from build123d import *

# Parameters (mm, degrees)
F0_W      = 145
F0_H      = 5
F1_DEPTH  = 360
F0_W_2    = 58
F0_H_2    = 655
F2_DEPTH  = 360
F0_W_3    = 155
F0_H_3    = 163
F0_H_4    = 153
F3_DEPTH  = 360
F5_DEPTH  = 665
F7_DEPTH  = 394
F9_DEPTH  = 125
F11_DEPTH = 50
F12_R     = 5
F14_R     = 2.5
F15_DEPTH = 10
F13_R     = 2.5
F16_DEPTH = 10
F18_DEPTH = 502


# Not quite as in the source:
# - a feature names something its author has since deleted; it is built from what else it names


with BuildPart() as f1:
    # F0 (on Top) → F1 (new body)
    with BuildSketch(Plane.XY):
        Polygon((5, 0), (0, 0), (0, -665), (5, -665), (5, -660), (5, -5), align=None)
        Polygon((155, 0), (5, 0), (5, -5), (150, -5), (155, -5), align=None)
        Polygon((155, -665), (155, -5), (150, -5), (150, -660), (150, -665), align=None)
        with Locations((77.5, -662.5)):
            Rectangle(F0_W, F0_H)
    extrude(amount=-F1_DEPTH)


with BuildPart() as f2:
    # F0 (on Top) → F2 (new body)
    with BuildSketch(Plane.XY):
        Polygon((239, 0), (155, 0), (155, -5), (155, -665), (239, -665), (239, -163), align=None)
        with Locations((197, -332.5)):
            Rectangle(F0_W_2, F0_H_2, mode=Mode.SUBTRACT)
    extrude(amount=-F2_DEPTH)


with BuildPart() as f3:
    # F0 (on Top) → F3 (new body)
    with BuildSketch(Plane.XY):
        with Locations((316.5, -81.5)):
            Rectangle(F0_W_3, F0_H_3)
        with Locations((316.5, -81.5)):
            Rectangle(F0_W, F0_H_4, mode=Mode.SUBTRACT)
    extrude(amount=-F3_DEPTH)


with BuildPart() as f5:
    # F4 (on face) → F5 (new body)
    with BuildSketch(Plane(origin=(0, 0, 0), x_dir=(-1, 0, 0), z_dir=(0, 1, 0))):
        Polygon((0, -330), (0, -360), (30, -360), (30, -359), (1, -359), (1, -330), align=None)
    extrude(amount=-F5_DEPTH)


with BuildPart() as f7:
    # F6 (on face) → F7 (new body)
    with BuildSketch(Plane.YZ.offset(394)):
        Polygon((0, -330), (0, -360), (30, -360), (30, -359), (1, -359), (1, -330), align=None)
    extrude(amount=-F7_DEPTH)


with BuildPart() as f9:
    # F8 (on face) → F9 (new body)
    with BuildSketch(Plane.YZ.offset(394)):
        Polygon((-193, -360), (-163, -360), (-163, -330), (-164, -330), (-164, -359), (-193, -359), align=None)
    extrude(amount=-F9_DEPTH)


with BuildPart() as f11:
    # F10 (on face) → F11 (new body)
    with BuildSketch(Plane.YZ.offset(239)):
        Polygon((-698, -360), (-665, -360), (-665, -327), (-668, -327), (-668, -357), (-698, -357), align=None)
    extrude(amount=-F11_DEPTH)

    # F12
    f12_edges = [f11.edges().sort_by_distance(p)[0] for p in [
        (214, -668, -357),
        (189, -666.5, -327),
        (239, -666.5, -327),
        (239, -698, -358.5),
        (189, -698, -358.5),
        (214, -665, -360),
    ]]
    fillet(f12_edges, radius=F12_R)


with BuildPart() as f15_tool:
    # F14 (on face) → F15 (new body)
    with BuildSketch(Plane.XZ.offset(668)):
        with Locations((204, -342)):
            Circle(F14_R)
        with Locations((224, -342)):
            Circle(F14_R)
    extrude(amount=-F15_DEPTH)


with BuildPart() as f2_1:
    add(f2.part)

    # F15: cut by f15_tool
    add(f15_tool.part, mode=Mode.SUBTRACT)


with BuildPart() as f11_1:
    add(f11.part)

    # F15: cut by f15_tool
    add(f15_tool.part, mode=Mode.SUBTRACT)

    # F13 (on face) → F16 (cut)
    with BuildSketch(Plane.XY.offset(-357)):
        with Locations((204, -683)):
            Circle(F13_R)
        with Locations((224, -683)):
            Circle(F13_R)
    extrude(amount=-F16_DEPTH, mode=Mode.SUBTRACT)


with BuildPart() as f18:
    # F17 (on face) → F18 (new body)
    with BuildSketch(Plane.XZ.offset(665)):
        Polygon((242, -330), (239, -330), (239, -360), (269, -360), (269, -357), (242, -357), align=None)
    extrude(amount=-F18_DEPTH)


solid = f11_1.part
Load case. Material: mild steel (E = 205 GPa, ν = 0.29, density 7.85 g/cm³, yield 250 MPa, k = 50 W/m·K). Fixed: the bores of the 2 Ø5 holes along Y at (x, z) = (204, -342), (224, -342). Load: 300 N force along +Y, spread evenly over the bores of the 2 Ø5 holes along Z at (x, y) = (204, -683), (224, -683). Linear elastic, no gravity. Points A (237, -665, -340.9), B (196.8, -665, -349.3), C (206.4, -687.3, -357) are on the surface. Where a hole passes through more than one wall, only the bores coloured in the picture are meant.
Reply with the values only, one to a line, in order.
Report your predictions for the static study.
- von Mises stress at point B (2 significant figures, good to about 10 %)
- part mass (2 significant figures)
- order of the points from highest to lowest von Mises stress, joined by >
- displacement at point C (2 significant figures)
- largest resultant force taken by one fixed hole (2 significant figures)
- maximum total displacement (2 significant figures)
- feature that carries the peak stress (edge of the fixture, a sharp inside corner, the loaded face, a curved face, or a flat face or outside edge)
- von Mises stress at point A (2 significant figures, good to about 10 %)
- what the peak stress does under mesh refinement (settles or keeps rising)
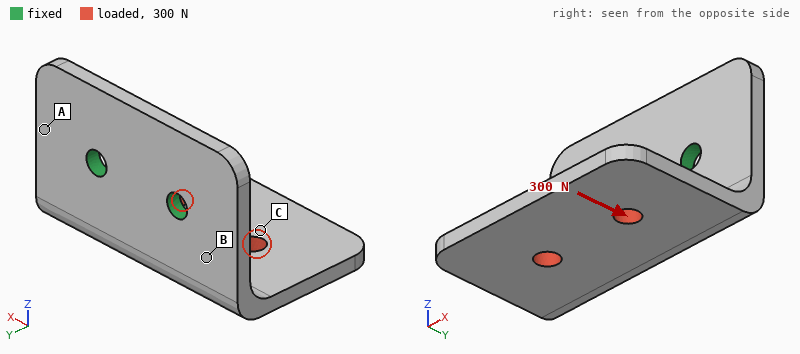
31 MPa
72 g
B > A > C
37 µm
150 N
55 µm
edge of the fixture
18 MPa
keeps rising
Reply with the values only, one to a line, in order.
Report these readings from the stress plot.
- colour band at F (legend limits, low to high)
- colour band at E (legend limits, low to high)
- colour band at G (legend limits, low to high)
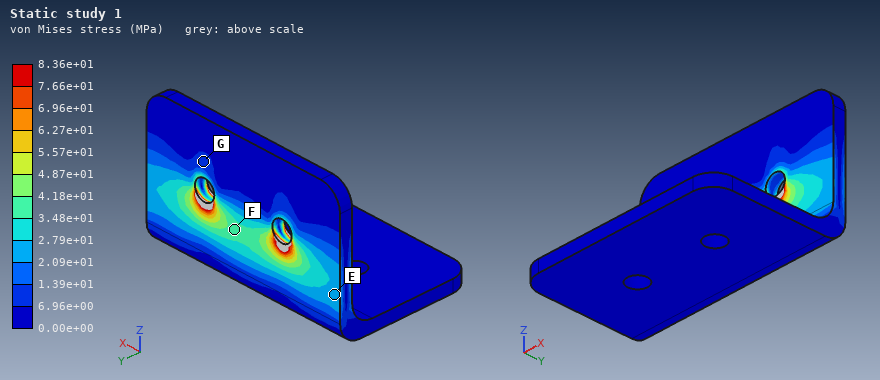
3.48e+01 to 4.18e+01 MPa
2.09e+01 to 2.79e+01 MPa
6.96e+00 to 1.39e+01 MPa
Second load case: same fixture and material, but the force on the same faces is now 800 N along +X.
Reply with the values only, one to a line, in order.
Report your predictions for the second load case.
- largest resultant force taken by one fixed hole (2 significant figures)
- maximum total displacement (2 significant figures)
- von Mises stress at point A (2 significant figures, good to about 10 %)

830 N
76 µm
48 MPa
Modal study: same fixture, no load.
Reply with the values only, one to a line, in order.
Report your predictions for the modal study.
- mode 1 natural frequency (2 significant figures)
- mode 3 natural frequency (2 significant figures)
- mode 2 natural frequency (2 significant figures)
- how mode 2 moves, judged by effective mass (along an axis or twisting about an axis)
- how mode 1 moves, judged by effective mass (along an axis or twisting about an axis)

1600 Hz
4800 Hz
2700 Hz
along X
along Z
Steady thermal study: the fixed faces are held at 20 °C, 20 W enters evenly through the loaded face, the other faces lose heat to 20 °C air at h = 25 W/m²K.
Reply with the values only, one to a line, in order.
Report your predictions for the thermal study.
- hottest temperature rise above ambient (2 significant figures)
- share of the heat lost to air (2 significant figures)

75 K
27 %
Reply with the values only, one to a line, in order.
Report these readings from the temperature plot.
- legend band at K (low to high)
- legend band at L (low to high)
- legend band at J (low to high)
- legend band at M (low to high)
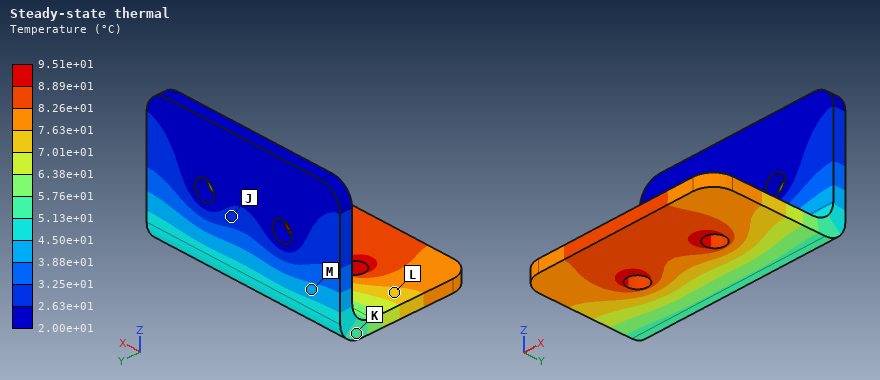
5.13e+01 to 5.76e+01 °C
7.01e+01 to 7.63e+01 °C
2.63e+01 to 3.25e+01 °C
3.88e+01 to 4.50e+01 °C
